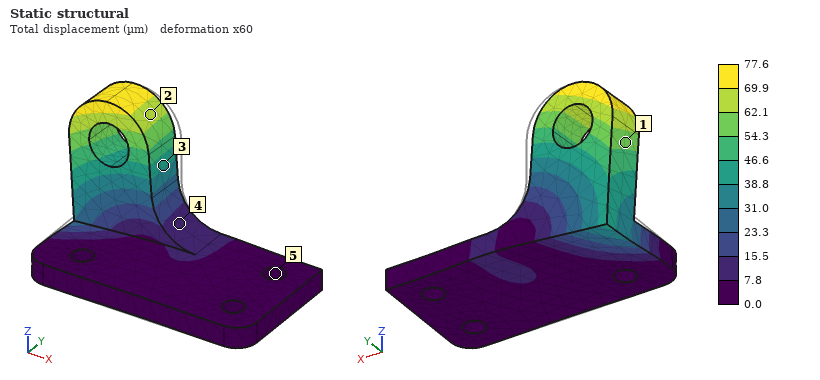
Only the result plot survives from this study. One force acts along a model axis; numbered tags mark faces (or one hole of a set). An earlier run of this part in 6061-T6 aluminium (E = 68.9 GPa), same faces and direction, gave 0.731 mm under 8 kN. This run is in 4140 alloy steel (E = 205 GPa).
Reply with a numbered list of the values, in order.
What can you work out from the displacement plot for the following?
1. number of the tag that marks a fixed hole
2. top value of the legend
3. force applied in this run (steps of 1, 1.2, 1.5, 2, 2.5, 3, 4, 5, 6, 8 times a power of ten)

1. 5
2. 77.6 µm
3. 2.5 kN
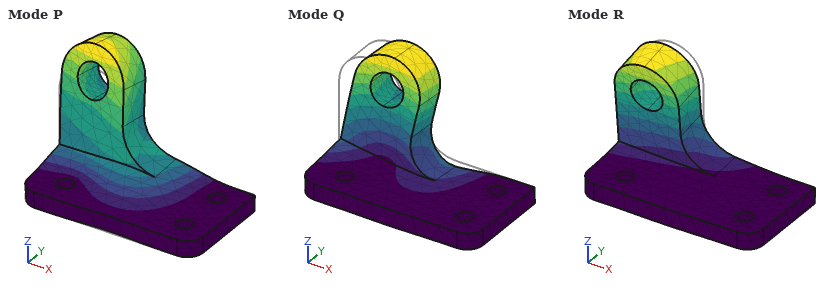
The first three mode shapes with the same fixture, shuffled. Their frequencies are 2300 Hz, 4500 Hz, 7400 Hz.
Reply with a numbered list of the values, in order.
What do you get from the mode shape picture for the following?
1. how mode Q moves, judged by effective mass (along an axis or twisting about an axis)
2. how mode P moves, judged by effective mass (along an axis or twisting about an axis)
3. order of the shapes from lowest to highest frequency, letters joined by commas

1. along X
2. along Z
3. R, Q, P
